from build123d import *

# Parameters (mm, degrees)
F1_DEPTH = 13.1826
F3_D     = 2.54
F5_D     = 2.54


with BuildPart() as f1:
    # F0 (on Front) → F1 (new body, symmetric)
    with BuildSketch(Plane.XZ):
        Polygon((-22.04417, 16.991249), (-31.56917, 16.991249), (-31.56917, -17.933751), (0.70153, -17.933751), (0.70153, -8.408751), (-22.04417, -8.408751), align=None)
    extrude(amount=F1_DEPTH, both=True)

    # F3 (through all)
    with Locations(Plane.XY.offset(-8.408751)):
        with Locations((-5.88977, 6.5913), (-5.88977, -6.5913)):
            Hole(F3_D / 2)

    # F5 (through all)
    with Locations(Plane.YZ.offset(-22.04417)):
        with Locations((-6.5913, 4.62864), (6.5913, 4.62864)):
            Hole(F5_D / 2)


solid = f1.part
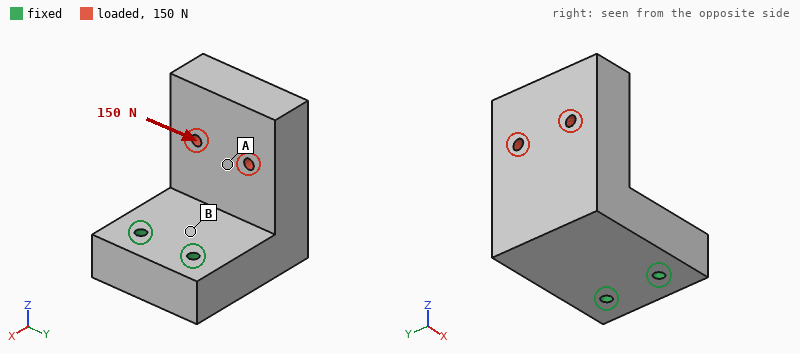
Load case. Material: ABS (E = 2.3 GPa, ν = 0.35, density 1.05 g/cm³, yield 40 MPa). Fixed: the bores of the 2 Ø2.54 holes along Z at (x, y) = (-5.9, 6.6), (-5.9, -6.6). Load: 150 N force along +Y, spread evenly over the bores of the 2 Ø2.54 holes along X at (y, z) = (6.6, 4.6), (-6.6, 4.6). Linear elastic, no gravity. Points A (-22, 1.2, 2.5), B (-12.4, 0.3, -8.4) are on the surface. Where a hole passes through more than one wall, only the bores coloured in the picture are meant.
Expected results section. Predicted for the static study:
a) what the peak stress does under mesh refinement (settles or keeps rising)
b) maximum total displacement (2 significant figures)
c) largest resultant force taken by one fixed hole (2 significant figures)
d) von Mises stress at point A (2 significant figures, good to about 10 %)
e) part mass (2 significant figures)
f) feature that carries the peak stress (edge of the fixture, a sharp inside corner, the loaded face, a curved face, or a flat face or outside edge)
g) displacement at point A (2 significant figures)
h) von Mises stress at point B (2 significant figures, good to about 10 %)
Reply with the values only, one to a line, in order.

keeps rising
0.30 mm
260 N
1.7 MPa
15 g
edge of the fixture
0.16 mm
6.7 MPa
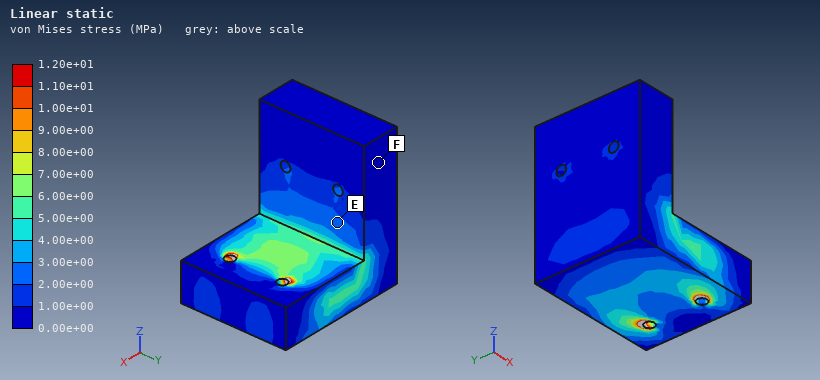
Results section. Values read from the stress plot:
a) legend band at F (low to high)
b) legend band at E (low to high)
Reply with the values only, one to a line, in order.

0.00e+00 to 1.00e+00 MPa
2.00e+00 to 3.00e+00 MPa
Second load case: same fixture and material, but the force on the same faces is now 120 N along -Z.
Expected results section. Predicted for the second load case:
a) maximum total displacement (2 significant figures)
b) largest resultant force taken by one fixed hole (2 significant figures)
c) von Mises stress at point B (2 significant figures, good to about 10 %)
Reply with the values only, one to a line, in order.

0.26 mm
60 N
3.5 MPa
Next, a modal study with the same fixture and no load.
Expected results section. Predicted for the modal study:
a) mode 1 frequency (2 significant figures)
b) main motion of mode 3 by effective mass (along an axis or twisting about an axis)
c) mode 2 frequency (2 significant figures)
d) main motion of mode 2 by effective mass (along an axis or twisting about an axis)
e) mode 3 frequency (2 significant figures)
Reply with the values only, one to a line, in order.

1100 Hz
along Z
1600 Hz
along Y
3000 Hz
